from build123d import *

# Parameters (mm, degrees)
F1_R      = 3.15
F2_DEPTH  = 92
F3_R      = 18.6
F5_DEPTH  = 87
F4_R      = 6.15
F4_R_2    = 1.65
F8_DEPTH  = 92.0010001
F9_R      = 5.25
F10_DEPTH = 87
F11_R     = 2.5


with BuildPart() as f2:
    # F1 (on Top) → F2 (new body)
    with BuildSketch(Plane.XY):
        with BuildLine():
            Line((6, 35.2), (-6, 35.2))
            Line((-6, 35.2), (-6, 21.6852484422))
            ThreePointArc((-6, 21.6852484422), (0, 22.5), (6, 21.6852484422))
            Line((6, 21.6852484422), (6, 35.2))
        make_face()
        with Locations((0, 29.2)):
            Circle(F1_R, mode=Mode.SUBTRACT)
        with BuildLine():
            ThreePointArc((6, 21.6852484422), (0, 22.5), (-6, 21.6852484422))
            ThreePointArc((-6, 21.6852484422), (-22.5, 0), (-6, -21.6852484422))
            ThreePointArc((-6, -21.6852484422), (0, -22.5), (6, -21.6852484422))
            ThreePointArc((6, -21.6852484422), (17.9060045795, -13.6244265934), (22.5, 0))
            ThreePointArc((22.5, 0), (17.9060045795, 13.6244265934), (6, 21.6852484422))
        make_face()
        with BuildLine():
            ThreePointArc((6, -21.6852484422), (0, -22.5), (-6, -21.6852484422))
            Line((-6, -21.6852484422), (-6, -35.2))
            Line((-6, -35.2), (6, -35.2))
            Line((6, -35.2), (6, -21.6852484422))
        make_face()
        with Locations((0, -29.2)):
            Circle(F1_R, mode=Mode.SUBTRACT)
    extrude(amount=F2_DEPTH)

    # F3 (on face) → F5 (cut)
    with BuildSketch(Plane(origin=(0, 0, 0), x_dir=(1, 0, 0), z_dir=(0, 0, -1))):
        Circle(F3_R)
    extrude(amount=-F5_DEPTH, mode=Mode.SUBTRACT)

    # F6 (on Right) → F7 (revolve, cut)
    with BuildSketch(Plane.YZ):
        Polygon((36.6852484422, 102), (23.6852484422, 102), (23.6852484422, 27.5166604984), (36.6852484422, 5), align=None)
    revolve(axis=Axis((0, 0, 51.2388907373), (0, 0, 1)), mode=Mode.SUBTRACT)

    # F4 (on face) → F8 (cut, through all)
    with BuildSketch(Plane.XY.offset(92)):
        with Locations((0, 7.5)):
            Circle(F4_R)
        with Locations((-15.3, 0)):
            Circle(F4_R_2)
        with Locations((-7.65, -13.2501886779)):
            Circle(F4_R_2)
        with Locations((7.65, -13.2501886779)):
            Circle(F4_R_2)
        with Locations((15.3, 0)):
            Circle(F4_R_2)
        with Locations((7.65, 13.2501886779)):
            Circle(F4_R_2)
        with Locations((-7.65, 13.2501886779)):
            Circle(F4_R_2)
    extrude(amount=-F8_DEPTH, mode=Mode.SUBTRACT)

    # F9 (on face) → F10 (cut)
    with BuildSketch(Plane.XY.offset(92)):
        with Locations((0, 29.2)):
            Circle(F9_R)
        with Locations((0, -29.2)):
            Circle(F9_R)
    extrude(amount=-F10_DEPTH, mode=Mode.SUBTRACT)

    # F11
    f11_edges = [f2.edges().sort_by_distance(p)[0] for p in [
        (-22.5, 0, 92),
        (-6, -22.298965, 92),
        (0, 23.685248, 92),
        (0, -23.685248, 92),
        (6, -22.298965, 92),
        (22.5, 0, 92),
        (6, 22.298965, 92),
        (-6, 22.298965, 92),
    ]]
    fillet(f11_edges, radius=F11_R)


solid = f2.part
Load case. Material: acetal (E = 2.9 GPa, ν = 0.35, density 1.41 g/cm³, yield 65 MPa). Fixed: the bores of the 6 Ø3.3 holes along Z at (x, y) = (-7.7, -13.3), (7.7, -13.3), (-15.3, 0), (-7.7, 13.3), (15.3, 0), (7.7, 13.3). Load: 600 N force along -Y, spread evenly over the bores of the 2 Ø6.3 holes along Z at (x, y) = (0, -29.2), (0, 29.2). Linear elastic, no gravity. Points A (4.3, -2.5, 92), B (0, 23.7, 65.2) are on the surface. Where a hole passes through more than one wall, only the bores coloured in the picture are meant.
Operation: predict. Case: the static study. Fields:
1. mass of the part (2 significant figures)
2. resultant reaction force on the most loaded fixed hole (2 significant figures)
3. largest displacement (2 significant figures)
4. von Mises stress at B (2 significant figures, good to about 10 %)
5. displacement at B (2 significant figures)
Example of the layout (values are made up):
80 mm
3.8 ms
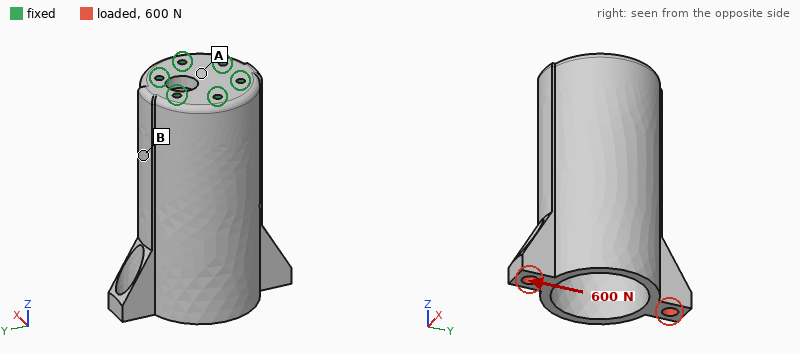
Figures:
79 g
790 N
1.4 mm
7.3 MPa
0.37 mm
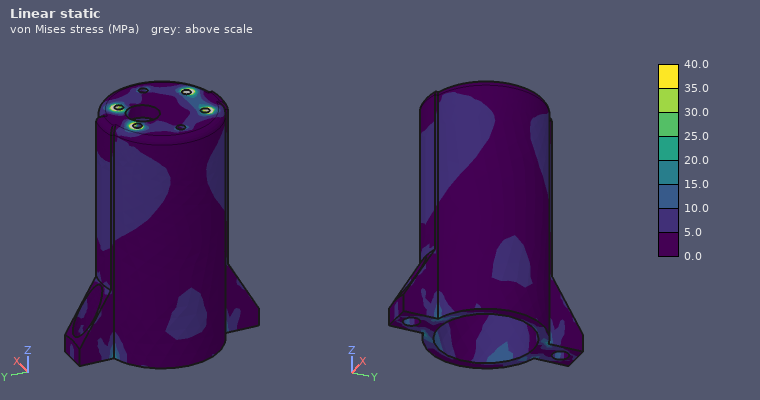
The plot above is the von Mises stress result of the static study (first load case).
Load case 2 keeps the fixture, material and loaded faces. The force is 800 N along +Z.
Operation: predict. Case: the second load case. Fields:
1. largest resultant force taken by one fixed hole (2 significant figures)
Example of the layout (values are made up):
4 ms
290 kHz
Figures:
140 N
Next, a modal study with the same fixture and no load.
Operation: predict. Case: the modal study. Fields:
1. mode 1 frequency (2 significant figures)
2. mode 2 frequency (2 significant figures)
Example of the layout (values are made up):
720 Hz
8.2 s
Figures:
700 Hz
710 Hz
